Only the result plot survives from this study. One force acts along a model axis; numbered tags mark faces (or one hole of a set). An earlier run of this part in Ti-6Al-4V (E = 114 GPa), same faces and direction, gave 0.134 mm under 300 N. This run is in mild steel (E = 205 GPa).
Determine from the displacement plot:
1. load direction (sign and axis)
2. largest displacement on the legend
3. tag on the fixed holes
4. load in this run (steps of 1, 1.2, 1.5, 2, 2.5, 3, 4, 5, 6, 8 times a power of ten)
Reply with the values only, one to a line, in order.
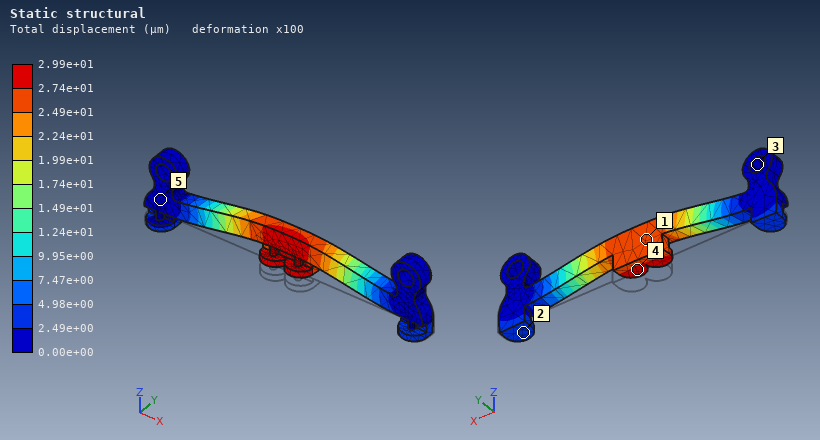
+Z
2.99e+01 µm
3
120 N
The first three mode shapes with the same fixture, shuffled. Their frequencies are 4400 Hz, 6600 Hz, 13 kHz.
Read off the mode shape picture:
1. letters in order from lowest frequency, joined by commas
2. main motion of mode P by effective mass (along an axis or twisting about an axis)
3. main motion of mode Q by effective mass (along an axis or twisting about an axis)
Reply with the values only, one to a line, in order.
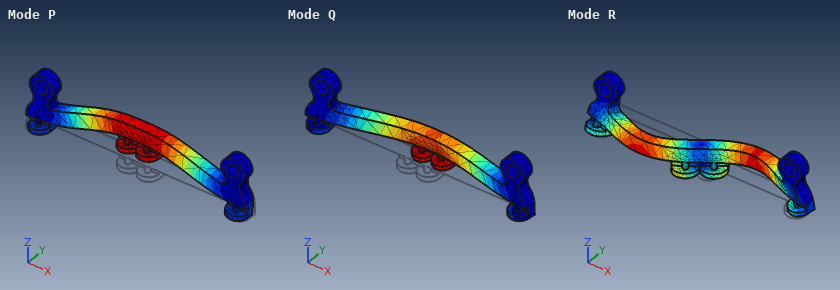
Q, P, R
along Z
along Y
